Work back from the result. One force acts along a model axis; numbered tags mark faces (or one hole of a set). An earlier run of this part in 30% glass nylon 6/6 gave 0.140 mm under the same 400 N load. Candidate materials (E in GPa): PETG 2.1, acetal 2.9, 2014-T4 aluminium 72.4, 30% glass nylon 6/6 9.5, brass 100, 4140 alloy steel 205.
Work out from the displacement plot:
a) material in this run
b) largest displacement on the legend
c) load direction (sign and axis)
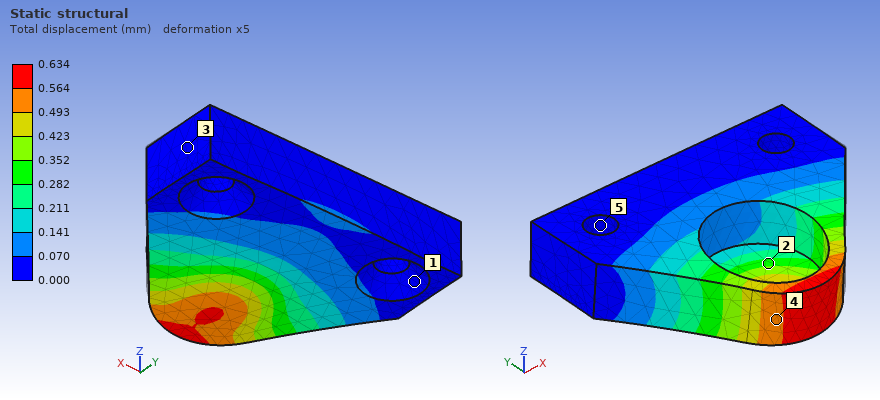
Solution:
PETG
0.634 mm
-Z
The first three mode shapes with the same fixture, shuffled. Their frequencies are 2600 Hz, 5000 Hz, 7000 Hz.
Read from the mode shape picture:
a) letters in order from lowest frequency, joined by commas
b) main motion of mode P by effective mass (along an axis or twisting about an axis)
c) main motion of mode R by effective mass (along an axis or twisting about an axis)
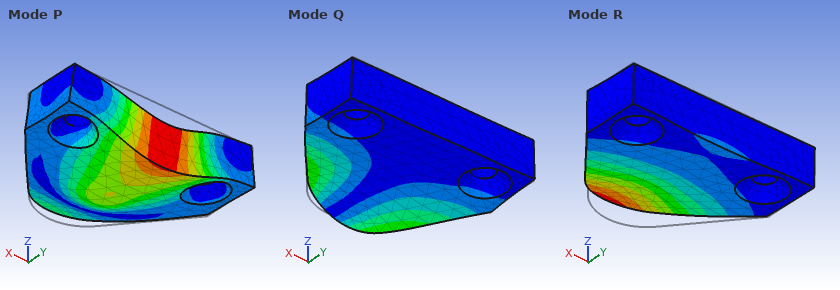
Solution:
R, Q, P
along Z
along Z
